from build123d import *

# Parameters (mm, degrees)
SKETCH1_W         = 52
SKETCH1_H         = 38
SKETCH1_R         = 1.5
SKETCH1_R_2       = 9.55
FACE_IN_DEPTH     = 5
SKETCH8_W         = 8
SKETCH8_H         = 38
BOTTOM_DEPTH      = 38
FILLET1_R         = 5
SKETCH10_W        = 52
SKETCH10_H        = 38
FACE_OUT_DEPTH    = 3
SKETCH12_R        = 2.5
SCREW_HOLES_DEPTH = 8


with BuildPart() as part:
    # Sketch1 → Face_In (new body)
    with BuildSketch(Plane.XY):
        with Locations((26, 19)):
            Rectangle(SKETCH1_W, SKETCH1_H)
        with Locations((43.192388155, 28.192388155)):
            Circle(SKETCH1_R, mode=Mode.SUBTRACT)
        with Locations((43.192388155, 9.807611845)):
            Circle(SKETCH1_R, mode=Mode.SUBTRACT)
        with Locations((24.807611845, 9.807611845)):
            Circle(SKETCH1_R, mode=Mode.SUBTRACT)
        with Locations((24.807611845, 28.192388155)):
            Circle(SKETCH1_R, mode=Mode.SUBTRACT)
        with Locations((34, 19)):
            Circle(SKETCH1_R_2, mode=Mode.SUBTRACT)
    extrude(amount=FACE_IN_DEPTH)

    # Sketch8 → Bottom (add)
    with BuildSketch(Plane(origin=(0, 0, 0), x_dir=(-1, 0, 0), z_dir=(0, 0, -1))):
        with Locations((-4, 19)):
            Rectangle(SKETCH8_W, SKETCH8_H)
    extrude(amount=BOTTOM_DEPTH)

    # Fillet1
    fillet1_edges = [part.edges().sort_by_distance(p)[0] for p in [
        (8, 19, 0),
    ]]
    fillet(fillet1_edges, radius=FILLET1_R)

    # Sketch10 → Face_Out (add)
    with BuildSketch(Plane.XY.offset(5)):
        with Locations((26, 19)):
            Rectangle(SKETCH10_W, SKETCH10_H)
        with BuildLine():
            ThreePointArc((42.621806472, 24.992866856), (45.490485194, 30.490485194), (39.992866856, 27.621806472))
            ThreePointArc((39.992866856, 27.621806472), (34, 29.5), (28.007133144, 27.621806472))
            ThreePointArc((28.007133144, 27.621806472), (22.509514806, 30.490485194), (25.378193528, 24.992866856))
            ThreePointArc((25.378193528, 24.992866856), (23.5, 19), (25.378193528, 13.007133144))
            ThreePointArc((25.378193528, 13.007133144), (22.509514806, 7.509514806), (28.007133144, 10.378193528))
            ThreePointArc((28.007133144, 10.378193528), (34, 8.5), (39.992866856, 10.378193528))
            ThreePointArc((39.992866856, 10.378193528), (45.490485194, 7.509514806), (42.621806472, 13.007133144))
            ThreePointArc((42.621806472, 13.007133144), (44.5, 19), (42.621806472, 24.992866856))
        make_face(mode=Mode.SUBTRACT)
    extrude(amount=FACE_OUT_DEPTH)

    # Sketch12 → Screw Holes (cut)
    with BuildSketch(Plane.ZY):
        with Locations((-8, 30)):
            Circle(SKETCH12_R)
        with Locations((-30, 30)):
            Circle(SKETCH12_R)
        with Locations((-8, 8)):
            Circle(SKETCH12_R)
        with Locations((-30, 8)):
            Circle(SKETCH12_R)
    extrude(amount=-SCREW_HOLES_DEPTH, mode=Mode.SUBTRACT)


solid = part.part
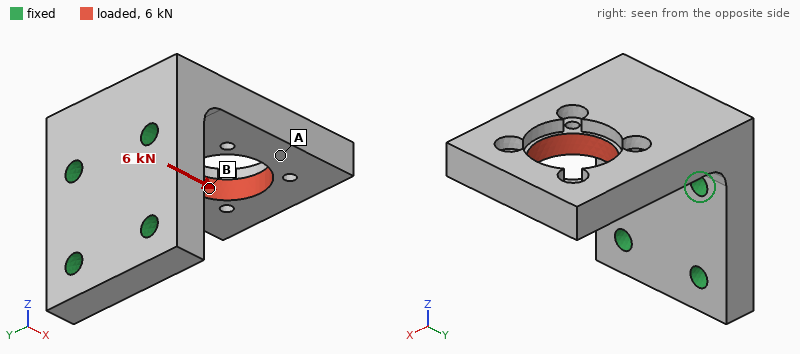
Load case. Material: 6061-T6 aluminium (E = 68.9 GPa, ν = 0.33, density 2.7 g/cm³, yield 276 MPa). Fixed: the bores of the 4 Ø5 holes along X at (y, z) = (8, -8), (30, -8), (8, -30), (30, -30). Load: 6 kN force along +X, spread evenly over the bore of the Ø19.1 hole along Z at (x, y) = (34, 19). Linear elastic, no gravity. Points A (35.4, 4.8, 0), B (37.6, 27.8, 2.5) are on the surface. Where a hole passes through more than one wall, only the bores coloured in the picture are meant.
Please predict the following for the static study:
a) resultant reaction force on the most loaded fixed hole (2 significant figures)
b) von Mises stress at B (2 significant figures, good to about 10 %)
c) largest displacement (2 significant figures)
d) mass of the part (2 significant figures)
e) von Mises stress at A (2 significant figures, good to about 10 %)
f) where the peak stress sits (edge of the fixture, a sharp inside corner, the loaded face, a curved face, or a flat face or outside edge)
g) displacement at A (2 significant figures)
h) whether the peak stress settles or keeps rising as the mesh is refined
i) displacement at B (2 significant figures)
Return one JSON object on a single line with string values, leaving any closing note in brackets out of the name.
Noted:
{"resultant reaction force on the most loaded fixed hole": "3.3 kN", "von Mises stress at B": "79 MPa", "largest displacement": "91 µm", "mass of the part": "65 g", "von Mises stress at A": "32 MPa", "where the peak stress sits": "edge of the fixture", "displacement at A": "74 µm", "whether the peak stress settles or keeps rising as the mesh is refined": "keeps rising", "displacement at B": "80 µm"}
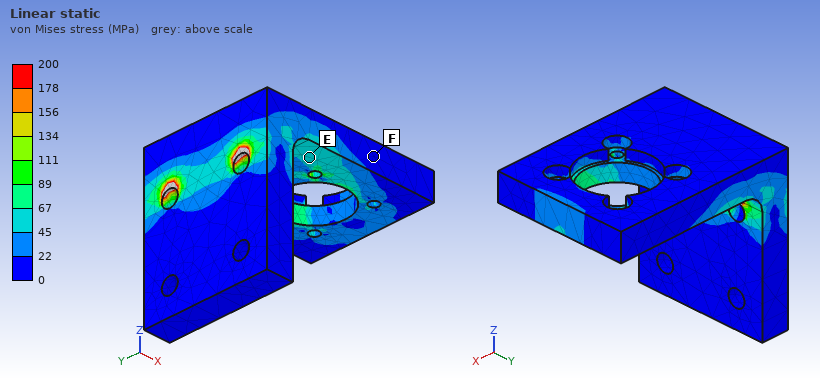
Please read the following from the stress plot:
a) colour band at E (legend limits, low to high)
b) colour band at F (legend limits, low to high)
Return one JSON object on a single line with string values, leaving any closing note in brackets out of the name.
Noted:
{"colour band at E": "45 to 67 MPa", "colour band at F": "0 to 22 MPa"}
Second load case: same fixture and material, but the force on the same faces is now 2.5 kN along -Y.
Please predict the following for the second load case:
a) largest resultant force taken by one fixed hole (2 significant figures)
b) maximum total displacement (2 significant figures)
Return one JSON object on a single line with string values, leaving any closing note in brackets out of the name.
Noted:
{"largest resultant force taken by one fixed hole": "3.2 kN", "maximum total displacement": "0.13 mm"}
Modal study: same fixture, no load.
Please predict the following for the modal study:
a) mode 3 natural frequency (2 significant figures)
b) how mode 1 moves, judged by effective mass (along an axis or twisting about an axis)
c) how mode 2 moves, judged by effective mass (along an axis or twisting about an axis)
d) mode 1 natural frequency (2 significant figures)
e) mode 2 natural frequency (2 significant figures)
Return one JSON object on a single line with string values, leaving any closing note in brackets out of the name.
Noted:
{"mode 3 natural frequency": "6100 Hz", "how mode 1 moves, judged by effective mass": "along Z", "how mode 2 moves, judged by effective mass": "along Y", "mode 1 natural frequency": "2500 Hz", "mode 2 natural frequency": "5300 Hz"}
